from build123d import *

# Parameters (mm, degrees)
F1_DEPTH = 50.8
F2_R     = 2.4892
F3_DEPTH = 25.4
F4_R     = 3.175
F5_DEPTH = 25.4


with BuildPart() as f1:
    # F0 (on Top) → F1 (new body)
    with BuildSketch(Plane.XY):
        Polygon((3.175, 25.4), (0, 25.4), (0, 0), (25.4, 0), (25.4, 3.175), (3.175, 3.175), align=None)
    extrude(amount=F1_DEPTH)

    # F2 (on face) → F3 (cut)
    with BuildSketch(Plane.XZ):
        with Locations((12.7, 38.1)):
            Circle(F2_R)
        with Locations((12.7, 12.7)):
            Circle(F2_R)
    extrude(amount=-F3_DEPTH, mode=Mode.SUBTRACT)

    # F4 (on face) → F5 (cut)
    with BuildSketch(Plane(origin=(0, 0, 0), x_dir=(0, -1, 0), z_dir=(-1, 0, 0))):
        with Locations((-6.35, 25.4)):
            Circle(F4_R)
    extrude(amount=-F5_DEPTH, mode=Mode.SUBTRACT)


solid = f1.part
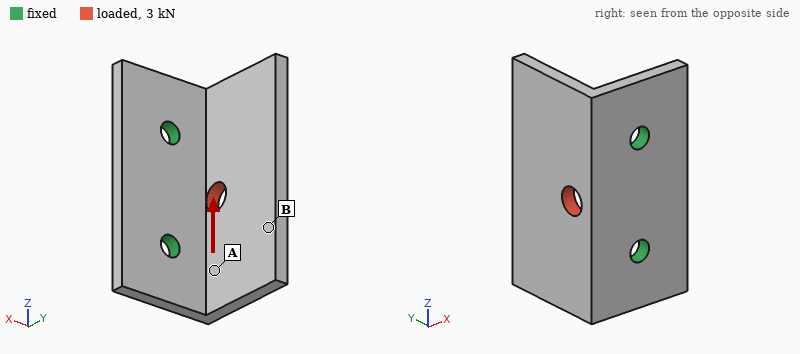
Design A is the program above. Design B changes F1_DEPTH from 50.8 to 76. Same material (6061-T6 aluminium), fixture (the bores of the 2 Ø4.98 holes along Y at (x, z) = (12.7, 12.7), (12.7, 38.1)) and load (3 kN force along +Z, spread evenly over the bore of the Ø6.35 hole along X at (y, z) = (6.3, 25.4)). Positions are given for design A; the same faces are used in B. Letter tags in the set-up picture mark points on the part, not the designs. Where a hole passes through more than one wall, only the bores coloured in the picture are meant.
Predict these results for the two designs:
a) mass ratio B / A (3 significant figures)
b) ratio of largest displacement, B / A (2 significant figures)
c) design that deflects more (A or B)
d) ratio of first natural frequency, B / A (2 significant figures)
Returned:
1.51
1.4
B
0.82
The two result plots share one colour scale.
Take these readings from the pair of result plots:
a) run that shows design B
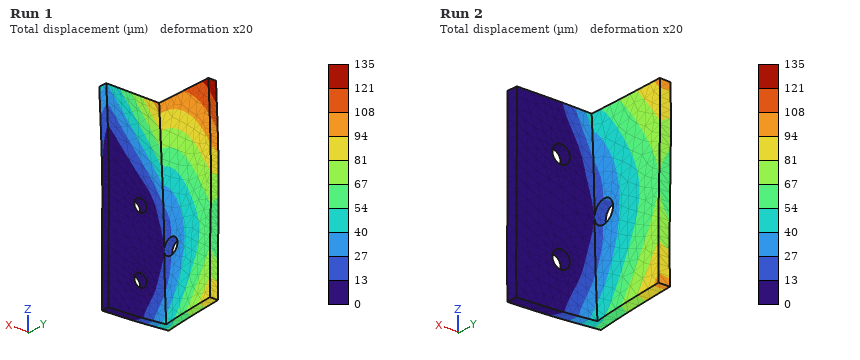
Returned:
Run 1
